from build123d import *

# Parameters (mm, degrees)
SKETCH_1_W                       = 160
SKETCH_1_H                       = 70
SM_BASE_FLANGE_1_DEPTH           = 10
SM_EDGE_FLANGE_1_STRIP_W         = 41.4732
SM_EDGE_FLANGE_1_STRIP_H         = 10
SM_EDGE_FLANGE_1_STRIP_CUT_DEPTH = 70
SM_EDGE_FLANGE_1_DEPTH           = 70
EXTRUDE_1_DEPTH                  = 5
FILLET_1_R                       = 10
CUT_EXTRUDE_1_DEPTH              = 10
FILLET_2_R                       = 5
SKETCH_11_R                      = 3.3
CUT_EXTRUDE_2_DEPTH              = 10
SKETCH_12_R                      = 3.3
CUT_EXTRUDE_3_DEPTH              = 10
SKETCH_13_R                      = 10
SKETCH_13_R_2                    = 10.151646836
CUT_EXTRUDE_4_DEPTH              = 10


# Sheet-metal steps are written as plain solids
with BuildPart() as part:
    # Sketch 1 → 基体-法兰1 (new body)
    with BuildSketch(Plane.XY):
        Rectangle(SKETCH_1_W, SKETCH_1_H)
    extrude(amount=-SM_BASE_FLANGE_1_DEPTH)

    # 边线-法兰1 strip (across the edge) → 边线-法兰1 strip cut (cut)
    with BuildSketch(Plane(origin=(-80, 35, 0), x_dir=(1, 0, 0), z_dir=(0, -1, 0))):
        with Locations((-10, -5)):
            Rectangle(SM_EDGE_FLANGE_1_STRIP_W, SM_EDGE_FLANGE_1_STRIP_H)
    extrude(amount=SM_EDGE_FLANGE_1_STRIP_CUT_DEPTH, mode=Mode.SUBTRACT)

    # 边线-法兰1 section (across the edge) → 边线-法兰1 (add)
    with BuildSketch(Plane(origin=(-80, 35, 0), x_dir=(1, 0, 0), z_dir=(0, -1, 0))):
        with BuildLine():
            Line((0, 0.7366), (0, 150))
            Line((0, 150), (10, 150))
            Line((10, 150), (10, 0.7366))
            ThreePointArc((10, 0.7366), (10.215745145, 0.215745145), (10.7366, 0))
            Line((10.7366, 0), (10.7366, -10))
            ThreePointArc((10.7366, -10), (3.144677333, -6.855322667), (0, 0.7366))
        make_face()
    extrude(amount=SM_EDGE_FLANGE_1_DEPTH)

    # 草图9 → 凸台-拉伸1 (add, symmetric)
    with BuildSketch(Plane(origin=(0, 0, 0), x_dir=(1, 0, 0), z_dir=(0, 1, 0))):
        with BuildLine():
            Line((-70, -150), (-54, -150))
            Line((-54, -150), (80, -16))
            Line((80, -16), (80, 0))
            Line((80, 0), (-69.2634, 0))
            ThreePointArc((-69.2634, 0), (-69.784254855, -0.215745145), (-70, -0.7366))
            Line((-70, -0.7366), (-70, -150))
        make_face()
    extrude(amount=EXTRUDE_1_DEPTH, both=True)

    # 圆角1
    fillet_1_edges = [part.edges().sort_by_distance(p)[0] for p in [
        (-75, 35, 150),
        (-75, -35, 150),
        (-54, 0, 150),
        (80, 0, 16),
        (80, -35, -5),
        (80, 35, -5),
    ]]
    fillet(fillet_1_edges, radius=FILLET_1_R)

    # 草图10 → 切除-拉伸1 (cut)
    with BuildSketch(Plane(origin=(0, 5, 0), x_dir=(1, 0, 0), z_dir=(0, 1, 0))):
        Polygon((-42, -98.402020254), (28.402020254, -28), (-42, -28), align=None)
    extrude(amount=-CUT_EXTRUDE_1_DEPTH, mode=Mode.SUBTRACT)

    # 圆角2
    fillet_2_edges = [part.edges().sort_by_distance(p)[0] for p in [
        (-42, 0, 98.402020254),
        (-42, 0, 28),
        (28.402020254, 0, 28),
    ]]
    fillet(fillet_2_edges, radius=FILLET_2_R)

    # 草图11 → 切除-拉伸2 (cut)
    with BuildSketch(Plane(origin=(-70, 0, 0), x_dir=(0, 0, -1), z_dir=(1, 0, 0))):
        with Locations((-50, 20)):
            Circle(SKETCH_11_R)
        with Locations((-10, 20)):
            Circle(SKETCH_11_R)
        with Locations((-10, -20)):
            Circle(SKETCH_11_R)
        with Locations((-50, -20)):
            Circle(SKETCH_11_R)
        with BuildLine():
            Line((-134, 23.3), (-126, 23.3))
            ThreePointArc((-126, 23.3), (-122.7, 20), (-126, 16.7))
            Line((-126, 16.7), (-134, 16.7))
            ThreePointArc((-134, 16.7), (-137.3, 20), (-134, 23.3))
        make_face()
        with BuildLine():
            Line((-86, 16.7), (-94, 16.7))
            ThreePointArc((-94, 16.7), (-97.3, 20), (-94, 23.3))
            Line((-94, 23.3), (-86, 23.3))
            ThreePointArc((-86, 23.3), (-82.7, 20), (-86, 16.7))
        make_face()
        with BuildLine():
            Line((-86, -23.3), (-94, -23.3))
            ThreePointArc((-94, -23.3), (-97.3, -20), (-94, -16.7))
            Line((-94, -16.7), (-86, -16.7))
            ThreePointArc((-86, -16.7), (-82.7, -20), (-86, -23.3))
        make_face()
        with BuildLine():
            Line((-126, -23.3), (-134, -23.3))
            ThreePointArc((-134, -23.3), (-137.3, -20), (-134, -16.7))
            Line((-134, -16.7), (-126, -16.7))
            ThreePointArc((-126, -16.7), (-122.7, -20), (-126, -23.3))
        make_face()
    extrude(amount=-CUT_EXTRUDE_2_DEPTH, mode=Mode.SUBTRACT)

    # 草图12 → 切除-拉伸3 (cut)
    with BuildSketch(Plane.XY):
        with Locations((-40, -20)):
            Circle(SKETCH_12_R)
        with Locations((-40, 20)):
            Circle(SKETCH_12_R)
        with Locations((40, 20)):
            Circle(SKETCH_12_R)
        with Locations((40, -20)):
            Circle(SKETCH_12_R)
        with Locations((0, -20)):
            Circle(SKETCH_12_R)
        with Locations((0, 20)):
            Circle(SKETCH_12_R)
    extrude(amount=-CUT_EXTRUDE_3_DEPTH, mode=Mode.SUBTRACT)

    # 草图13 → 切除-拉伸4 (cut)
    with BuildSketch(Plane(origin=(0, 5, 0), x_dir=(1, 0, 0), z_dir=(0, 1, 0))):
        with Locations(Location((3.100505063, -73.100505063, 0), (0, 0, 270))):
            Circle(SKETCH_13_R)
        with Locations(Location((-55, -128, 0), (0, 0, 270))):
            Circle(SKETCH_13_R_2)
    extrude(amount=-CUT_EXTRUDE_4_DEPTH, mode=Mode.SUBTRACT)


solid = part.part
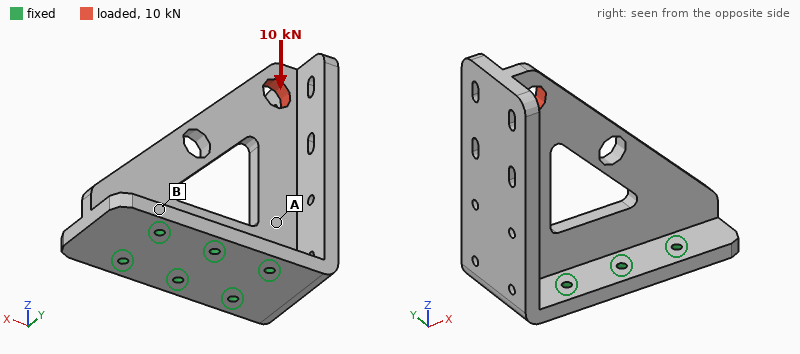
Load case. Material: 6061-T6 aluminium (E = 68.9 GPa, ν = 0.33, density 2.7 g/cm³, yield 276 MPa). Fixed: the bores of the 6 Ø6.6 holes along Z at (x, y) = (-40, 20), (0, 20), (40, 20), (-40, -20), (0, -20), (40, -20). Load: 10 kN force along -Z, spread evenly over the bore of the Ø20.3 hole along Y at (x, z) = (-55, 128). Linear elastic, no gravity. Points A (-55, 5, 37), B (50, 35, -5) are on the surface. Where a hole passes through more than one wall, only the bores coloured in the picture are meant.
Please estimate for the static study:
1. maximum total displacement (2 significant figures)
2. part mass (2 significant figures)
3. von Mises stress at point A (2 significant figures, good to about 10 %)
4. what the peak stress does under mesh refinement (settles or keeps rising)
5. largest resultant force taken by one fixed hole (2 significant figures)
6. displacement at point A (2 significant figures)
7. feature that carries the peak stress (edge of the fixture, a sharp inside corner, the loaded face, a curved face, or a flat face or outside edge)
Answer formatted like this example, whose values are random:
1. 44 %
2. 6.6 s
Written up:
1. 0.13 mm
2. 840 g
3. 21 MPa
4. keeps rising
5. 5.5 kN
6. 0.068 mm
7. edge of the fixture
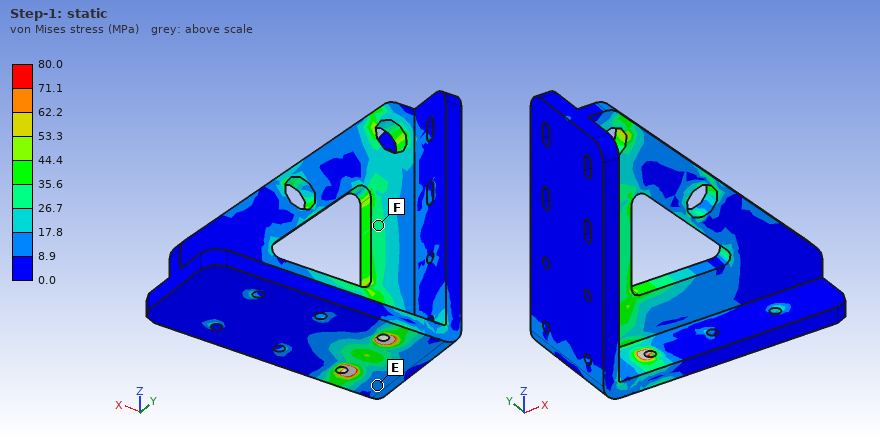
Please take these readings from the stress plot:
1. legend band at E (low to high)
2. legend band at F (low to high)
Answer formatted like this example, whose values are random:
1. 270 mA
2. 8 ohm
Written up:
1. 8.9 to 17.8 MPa
2. 26.7 to 35.6 MPa
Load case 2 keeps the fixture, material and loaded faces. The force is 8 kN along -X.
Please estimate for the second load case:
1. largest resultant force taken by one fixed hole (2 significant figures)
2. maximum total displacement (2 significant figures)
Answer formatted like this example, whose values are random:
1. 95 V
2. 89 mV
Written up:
1. 6.1 kN
2. 0.37 mm
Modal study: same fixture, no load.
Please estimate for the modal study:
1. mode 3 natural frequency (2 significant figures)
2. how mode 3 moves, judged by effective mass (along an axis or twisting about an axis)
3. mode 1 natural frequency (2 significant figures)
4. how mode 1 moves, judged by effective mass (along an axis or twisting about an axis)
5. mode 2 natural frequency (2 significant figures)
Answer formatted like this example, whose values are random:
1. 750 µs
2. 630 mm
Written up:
1. 1600 Hz
2. along X
3. 640 Hz
4. along Y
5. 1500 Hz
